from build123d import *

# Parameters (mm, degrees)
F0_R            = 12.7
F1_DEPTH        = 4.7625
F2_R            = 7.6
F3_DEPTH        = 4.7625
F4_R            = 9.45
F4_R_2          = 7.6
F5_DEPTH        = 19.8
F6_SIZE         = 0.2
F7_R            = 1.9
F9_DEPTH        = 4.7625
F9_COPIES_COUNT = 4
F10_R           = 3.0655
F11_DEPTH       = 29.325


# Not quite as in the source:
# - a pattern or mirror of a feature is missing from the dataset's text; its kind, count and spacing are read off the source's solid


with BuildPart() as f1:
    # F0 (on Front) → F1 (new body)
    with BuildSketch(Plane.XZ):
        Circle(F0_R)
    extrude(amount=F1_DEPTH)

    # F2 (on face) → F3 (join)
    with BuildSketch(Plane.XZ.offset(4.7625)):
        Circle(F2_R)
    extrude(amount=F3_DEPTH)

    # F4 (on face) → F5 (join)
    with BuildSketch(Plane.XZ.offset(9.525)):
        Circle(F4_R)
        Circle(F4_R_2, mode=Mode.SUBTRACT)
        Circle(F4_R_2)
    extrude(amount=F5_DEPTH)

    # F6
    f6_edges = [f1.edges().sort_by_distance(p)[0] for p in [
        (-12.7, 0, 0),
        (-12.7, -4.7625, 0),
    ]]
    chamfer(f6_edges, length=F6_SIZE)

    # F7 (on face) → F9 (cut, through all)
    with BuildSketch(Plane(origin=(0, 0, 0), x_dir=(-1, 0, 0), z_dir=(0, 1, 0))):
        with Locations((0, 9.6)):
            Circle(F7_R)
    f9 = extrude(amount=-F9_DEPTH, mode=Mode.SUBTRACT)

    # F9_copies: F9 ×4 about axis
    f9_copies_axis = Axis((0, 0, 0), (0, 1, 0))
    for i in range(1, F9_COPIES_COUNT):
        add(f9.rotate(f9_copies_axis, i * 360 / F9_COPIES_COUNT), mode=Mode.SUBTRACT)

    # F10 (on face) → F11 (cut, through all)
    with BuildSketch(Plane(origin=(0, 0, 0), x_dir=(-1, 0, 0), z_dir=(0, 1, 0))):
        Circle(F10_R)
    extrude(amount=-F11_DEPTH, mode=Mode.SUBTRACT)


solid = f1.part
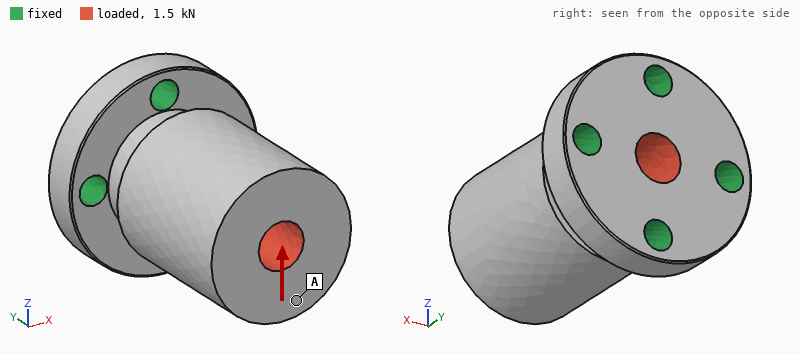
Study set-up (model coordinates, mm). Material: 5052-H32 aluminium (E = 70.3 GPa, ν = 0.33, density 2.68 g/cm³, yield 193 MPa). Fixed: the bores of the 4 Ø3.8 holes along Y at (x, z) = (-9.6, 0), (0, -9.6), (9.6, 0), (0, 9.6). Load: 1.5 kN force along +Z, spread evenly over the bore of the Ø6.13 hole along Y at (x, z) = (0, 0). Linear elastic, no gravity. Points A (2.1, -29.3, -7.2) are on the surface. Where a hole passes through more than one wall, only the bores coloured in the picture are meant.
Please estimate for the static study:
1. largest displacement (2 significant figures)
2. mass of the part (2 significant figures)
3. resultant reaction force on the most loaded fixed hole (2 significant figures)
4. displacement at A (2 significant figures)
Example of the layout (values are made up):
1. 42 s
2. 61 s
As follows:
1. 26 µm
2. 21 g
3. 1.1 kN
4. 25 µm
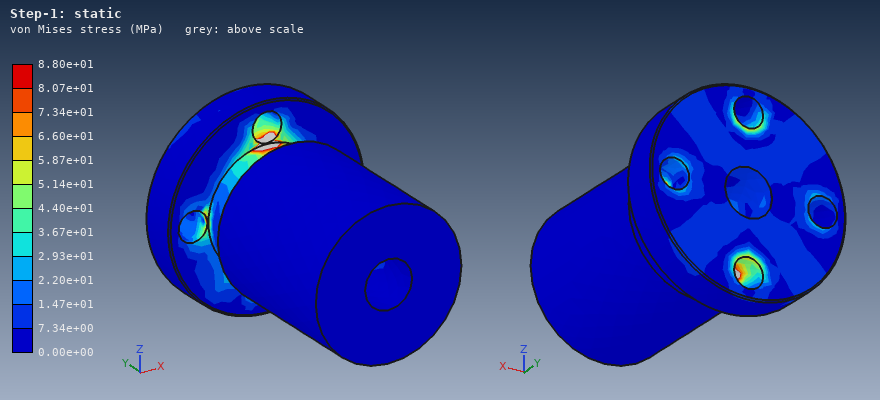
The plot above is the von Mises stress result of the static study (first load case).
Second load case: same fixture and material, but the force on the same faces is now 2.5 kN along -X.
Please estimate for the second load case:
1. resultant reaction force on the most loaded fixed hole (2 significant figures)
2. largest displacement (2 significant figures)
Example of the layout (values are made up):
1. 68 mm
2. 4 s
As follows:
1. 1.9 kN
2. 43 µm
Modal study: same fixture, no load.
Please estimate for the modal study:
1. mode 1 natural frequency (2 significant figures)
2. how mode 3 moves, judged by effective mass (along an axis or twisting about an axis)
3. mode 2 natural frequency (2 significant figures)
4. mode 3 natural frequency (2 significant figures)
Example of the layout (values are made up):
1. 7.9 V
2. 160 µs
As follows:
1. 10 kHz
2. twisting about Y
3. 10 kHz
4. 23 kHz
